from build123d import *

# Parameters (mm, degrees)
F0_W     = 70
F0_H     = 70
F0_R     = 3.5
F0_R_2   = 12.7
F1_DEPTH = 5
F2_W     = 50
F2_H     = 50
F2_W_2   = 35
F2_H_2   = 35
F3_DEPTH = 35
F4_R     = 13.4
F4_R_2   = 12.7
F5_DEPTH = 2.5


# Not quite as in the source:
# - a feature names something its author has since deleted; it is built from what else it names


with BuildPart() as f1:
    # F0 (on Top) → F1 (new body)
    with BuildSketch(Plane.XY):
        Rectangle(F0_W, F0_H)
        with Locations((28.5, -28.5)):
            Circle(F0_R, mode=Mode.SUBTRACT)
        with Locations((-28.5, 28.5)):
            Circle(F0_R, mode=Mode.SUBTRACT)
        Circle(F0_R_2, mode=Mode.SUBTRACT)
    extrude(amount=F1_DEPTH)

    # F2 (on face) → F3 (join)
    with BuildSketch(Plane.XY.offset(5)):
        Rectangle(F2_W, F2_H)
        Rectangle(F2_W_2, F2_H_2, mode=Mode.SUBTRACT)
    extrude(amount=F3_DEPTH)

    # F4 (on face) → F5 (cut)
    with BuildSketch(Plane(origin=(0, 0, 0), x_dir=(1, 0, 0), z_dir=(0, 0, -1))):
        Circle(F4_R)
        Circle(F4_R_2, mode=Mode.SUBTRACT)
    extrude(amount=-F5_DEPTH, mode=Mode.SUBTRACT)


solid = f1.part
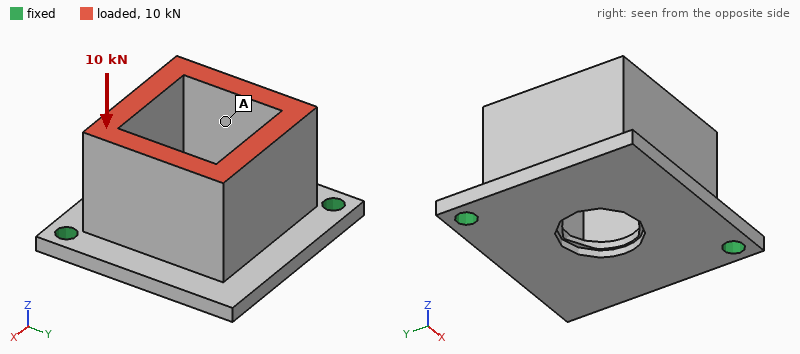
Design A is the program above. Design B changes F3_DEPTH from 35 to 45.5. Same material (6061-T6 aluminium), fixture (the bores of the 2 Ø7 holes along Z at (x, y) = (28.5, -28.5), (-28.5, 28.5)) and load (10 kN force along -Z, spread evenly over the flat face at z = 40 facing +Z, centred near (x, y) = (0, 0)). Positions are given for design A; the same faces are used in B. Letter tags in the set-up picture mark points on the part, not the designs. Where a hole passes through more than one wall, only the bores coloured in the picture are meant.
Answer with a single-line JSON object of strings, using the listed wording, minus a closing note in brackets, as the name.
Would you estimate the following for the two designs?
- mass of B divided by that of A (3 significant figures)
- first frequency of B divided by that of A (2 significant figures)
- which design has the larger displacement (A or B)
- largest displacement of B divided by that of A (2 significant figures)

{"mass of B divided by that of A": "1.20", "first frequency of B divided by that of A": "0.78", "which design has the larger displacement": "A", "largest displacement of B divided by that of A": "0.72"}
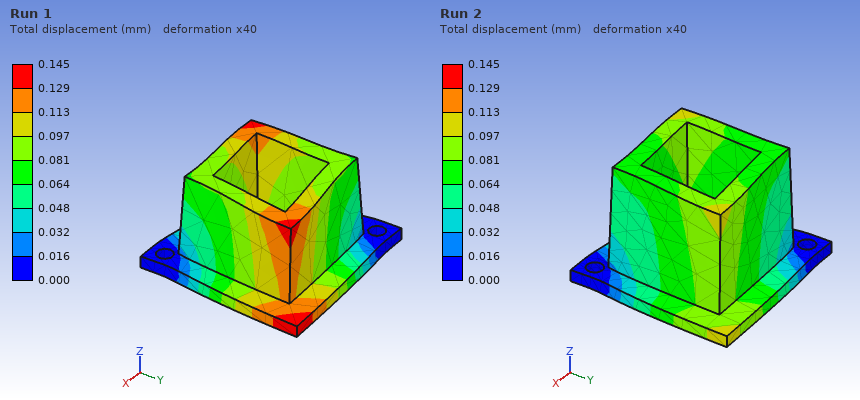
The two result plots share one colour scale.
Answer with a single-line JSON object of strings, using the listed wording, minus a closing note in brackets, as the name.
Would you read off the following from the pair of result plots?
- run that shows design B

{"run that shows design B": "Run 2"}
